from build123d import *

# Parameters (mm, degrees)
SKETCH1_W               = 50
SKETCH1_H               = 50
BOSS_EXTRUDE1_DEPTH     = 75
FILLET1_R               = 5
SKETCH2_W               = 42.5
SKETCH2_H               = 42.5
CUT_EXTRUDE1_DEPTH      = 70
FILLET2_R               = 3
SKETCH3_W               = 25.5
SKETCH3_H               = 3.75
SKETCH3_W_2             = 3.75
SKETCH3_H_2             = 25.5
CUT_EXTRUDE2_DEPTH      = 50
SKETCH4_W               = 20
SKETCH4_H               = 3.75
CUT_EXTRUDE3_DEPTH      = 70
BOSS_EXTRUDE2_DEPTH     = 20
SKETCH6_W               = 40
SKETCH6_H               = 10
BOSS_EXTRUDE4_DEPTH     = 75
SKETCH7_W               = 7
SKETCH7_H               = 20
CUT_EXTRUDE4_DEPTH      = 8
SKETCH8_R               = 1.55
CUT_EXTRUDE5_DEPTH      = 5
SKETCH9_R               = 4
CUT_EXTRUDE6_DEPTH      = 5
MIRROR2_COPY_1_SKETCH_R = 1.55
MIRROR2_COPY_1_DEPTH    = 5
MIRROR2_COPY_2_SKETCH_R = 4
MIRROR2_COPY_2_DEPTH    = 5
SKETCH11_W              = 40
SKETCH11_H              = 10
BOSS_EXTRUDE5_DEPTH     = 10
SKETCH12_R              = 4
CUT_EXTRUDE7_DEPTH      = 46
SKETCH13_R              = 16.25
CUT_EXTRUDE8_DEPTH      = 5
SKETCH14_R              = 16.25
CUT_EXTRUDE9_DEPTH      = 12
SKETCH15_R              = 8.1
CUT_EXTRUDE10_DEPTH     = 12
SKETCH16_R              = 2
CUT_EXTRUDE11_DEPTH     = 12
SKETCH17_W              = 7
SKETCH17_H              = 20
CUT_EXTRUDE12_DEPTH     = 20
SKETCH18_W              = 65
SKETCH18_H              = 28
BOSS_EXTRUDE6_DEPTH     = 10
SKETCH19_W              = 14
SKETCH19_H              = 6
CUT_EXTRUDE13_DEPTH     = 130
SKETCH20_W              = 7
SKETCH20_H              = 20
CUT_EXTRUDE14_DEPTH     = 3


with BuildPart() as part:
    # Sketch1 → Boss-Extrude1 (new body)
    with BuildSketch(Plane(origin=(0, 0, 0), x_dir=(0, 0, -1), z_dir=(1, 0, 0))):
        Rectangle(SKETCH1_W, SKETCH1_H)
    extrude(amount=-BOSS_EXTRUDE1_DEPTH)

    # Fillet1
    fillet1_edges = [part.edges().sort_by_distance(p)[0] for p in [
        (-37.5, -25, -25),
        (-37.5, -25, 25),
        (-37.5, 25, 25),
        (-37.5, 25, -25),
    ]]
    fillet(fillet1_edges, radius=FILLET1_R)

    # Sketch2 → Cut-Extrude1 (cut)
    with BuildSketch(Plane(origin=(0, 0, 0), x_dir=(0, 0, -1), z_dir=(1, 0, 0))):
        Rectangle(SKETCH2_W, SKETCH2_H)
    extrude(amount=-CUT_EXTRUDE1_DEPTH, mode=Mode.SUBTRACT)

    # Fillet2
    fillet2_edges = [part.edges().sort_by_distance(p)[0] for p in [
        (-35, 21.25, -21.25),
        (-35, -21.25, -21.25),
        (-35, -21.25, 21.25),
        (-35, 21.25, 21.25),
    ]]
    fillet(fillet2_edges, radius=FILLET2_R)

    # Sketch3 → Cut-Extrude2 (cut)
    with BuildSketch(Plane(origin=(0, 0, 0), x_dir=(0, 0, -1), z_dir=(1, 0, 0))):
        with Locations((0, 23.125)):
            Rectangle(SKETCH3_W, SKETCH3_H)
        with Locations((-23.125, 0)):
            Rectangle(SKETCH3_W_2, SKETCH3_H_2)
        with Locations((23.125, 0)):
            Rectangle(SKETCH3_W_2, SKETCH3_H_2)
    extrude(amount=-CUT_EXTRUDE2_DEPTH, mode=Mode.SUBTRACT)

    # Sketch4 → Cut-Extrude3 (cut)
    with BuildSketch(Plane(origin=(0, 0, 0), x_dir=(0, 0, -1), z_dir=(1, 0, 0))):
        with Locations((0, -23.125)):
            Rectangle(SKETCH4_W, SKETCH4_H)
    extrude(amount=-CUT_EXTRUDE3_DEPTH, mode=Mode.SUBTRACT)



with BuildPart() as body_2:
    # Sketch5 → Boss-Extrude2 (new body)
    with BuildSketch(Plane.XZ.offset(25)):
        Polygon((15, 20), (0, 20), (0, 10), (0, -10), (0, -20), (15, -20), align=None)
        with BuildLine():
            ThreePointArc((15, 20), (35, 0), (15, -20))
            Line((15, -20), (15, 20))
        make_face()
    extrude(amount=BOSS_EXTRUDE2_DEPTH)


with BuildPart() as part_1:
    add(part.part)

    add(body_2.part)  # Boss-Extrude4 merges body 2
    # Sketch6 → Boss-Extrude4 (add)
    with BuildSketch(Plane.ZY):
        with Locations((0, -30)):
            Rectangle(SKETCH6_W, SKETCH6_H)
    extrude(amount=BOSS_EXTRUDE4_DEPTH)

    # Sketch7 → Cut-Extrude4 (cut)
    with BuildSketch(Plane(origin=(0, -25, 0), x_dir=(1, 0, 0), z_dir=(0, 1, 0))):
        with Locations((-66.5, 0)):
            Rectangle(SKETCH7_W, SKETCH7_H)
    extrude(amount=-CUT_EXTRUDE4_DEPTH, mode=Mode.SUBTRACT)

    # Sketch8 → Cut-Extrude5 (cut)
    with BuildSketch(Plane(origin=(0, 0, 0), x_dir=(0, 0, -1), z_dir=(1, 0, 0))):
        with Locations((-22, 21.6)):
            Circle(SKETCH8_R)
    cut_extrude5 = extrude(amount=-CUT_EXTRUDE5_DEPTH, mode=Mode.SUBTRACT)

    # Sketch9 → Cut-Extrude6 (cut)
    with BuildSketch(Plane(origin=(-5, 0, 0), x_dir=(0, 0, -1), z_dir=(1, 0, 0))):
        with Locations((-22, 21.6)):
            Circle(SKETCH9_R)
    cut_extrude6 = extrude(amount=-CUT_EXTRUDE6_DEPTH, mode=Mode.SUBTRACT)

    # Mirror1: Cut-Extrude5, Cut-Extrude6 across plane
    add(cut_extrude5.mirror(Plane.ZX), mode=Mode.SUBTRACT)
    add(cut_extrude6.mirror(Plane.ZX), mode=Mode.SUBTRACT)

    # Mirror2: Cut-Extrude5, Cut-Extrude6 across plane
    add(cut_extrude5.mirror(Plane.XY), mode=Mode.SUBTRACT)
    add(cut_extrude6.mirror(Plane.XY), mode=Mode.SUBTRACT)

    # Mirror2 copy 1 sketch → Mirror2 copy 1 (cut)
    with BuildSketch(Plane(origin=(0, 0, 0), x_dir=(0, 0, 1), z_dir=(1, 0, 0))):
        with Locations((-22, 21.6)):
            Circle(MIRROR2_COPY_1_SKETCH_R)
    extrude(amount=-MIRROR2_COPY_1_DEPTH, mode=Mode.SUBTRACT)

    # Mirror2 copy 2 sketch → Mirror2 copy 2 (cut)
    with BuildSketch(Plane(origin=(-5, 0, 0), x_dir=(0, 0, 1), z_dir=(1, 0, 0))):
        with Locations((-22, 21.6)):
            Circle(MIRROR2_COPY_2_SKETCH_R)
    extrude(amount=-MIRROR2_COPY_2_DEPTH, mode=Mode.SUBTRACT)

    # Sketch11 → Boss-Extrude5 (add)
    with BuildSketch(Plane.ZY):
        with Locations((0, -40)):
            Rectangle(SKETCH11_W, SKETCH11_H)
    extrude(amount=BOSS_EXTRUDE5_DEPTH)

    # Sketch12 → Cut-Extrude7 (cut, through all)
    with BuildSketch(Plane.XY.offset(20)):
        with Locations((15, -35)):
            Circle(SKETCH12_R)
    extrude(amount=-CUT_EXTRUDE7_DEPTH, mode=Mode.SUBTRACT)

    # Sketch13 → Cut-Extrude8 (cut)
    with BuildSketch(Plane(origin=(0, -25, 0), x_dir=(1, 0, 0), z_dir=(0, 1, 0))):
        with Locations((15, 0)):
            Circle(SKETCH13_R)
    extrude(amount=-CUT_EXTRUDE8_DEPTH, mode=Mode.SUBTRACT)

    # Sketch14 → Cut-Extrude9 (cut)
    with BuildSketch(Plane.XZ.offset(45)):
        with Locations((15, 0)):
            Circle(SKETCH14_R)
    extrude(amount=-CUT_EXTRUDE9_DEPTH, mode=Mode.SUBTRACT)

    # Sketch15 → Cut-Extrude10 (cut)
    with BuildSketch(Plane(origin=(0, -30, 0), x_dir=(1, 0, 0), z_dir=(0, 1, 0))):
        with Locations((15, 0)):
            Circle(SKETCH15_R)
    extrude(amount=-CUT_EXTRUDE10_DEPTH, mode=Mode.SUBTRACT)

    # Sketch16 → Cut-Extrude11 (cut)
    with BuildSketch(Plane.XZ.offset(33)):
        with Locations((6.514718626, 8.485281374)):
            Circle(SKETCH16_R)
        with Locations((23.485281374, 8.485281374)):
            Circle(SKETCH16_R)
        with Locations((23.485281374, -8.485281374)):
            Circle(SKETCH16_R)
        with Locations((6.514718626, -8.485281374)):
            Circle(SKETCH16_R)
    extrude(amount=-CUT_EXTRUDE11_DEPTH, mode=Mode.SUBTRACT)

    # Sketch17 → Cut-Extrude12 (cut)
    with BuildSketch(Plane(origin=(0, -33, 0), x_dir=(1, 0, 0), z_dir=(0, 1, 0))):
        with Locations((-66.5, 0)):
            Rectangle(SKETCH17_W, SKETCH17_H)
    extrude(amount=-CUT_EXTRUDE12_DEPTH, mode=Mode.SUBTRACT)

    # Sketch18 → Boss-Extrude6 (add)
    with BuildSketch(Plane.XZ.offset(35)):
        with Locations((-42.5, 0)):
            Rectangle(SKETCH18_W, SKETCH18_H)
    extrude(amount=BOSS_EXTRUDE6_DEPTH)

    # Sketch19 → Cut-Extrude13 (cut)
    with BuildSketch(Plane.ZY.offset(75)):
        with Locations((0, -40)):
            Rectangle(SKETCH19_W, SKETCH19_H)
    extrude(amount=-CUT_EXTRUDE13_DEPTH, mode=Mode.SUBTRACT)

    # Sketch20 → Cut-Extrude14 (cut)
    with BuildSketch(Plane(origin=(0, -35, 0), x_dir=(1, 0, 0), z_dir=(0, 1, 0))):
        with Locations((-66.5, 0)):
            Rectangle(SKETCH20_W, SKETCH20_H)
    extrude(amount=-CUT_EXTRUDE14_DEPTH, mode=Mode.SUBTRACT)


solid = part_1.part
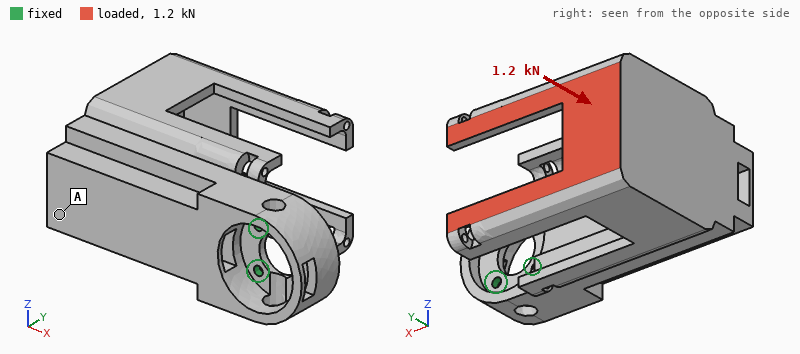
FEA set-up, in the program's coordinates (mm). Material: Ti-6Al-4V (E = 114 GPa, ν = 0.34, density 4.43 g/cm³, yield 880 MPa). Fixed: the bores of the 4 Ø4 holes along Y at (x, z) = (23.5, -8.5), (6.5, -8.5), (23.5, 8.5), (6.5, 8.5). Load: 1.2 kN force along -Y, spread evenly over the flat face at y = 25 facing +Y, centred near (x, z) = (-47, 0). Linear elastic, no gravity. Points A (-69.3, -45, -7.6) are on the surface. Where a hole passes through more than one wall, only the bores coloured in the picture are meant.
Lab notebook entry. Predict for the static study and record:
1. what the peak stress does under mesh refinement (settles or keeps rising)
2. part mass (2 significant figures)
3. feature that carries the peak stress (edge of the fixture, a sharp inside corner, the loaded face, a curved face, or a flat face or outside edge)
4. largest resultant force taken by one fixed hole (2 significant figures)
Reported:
keeps rising
410 g
edge of the fixture
1.9 kN
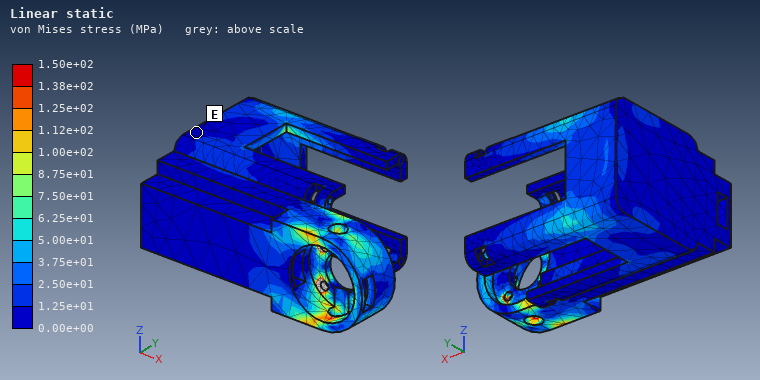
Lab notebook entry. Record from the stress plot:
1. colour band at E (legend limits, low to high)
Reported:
0.00e+00 to 1.25e+01 MPa
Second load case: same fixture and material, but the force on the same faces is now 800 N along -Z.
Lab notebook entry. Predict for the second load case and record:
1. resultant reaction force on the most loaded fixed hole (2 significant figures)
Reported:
2.0 kN
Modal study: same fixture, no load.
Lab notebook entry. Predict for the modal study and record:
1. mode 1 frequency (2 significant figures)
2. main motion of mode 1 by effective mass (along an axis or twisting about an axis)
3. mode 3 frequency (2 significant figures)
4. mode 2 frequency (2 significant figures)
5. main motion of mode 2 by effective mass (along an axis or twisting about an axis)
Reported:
600 Hz
along Y
1600 Hz
900 Hz
along Z
